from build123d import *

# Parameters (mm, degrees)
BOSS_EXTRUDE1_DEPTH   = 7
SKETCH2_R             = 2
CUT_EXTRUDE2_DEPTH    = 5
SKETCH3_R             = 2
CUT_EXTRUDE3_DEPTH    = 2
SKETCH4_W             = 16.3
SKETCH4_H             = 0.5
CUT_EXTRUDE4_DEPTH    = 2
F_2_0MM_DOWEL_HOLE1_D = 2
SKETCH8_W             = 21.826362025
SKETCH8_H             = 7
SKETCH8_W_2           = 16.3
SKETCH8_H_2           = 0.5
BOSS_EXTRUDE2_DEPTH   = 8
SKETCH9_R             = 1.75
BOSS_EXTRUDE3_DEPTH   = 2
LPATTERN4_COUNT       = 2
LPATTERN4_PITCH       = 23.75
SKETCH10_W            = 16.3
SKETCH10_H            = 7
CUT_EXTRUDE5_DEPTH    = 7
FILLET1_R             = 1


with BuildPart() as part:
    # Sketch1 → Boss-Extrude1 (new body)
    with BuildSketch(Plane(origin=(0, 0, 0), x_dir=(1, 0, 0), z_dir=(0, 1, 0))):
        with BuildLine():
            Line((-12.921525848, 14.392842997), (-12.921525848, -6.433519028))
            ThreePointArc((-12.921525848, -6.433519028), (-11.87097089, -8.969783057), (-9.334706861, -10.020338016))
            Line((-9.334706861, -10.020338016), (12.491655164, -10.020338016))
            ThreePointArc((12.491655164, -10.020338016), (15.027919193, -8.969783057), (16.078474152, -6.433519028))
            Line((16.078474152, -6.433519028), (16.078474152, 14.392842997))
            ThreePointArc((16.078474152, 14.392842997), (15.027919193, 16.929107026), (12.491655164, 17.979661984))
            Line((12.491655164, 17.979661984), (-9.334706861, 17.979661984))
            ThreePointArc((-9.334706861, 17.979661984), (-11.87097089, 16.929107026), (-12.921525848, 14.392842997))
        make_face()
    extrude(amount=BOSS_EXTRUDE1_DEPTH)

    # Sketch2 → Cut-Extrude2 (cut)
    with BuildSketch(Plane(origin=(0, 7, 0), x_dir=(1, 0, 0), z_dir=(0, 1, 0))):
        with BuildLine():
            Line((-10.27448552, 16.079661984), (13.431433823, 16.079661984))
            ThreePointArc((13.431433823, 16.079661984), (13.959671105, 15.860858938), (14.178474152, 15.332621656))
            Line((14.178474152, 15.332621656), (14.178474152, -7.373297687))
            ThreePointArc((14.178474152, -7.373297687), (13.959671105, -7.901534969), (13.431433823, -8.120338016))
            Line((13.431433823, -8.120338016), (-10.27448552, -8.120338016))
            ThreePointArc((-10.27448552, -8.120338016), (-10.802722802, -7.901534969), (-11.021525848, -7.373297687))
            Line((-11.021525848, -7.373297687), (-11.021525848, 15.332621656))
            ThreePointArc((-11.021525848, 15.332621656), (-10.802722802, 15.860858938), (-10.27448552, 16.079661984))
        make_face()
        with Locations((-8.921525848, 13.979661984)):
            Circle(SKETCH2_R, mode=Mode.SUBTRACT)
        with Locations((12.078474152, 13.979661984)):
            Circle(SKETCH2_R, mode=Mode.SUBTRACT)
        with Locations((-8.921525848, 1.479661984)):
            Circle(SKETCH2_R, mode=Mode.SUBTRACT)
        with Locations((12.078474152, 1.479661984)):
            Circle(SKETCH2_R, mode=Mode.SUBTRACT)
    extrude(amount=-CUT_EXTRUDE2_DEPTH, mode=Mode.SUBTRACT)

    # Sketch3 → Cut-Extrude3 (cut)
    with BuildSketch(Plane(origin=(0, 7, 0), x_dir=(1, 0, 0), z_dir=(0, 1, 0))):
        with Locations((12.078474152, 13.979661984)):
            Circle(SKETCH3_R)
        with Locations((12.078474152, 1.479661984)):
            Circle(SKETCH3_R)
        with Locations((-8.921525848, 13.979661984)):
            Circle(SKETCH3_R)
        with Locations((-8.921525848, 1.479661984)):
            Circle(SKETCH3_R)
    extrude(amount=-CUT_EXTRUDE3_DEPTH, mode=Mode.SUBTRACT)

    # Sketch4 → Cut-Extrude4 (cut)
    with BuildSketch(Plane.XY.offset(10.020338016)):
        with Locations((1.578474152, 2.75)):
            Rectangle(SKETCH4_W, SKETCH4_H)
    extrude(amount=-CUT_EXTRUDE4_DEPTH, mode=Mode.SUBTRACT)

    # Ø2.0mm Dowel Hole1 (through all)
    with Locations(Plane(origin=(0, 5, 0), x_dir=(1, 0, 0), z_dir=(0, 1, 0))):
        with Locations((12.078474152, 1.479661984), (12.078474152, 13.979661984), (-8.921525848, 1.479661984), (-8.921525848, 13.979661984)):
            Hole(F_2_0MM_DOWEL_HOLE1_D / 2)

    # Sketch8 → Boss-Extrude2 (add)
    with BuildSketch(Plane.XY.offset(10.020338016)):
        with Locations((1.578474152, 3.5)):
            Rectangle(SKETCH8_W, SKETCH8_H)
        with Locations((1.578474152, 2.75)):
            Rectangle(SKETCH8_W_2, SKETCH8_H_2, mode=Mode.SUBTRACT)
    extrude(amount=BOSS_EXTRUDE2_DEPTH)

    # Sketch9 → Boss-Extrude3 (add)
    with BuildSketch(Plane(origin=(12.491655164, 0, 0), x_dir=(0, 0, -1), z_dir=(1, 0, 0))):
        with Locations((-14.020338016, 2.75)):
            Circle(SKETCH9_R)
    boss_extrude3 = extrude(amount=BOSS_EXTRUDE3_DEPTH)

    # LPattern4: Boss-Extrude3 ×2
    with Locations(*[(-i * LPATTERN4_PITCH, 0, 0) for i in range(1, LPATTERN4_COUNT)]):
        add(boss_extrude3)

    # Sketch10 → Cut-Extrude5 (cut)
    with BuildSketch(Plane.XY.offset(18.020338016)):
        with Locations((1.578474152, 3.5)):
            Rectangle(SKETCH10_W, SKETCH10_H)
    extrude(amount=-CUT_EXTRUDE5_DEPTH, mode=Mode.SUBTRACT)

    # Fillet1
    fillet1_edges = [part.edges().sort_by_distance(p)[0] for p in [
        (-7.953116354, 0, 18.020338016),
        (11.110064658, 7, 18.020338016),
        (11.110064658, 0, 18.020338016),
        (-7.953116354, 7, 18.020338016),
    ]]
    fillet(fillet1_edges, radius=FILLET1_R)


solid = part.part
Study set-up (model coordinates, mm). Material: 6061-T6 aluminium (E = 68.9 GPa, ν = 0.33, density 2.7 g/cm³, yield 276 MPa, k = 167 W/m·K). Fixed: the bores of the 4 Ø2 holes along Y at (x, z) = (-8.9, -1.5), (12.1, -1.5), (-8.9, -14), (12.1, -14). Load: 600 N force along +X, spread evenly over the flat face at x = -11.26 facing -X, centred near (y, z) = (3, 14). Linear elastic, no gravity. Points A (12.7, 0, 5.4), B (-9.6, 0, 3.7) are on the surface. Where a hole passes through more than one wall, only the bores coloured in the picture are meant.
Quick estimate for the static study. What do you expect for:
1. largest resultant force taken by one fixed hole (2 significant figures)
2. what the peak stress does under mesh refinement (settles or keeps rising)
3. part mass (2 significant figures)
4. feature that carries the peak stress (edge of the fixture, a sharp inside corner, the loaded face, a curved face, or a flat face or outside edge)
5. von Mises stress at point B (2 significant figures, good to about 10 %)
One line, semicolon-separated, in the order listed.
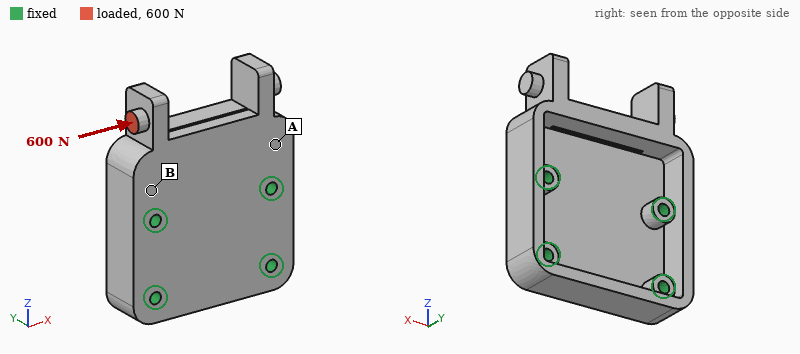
470 N; keeps rising; 8.3 g; a sharp inside corner; 35 MPa
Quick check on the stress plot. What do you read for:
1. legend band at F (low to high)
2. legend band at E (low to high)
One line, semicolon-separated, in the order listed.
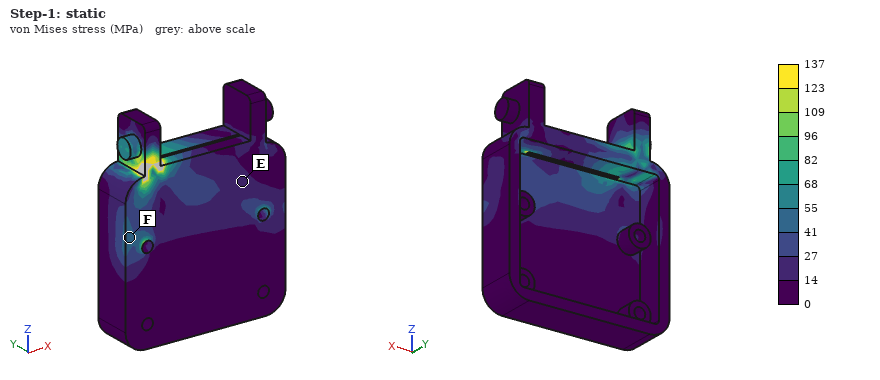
41 to 55 MPa; 14 to 27 MPa
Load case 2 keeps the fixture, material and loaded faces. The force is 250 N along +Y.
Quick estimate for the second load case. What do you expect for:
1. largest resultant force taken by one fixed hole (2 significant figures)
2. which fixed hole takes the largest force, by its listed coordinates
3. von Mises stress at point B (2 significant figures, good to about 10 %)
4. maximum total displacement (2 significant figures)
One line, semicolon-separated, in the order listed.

500 N; (-8.9, -1.5); 54 MPa; 0.14 mm
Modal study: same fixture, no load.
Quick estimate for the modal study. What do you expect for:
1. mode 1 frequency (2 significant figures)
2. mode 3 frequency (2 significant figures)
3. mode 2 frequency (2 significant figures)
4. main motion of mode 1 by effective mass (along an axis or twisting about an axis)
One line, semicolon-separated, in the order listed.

8100 Hz; 19 kHz; 11 kHz; along Y
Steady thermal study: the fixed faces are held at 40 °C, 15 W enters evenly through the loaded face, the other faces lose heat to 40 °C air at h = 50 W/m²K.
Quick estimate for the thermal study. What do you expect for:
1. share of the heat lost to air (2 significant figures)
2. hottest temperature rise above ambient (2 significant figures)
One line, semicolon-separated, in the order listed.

8.6 %; 68 K
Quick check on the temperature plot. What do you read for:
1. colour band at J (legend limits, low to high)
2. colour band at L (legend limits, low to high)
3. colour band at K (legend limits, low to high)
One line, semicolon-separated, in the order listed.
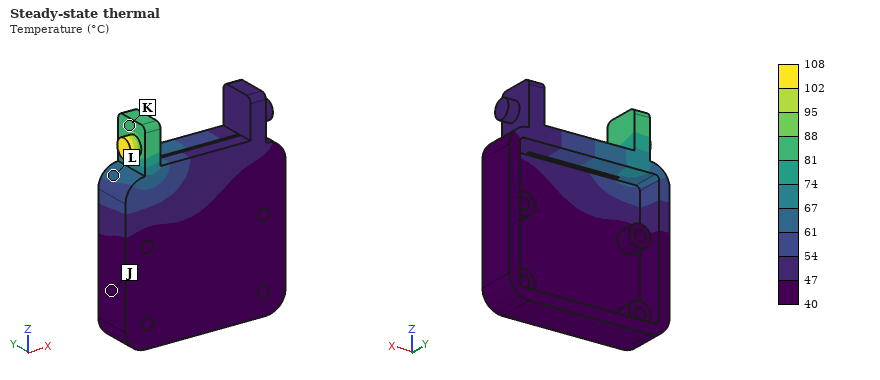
40 to 47 °C; 61 to 67 °C; 81 to 88 °C
